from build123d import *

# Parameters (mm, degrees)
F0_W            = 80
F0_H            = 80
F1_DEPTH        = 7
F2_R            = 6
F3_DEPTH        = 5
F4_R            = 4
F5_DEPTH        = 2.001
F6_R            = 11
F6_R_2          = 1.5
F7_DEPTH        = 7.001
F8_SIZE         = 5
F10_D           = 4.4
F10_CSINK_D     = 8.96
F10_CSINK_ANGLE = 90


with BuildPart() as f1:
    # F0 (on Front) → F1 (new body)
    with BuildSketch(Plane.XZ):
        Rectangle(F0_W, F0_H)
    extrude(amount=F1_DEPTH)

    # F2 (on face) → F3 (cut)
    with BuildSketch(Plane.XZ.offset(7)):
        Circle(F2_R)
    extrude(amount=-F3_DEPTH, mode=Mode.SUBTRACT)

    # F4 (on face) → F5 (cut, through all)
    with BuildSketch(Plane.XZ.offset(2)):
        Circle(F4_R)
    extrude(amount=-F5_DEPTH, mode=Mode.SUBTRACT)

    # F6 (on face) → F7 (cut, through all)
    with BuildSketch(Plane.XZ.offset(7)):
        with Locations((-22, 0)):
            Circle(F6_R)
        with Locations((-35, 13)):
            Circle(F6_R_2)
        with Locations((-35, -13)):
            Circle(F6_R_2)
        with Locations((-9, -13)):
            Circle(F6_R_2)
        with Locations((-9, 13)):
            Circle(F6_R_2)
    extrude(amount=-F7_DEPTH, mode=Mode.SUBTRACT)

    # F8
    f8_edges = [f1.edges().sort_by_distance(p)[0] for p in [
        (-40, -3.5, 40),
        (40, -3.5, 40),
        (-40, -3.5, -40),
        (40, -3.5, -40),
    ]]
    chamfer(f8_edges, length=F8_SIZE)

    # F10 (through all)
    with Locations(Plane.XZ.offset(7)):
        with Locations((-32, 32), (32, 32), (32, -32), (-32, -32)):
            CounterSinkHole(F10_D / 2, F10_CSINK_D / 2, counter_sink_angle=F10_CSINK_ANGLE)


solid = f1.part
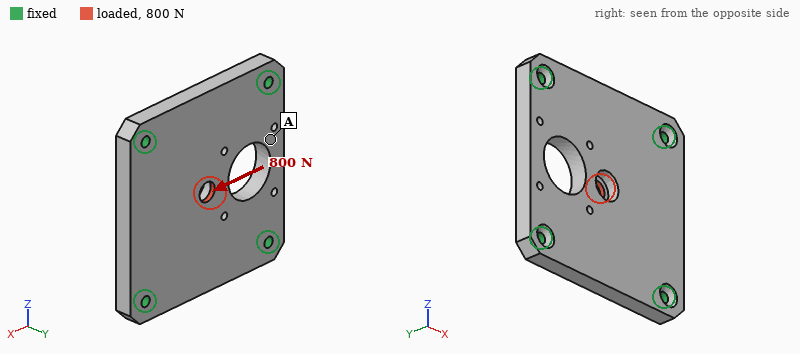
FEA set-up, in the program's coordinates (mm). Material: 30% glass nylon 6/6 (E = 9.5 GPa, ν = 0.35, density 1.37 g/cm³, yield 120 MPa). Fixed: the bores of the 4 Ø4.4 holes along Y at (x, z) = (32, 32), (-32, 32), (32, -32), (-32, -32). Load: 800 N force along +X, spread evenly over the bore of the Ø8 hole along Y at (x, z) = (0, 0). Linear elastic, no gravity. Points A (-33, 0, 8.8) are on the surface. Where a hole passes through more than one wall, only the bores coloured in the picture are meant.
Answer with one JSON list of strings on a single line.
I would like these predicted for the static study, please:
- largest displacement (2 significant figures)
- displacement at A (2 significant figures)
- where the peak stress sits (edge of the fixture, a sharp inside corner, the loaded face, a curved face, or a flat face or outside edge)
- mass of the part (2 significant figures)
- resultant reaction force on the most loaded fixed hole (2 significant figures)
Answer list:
["27 µm", "8.8 µm", "a sharp inside corner", "55 g", "230 N"]
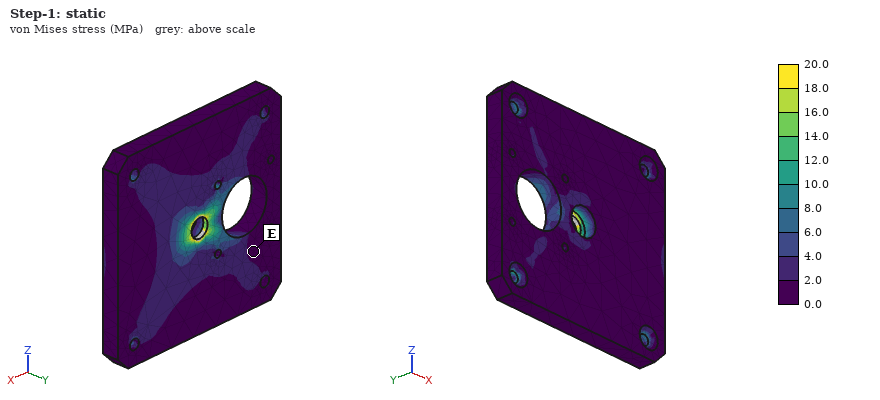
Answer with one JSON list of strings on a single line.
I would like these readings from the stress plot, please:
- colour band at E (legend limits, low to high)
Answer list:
["0.0 to 2.0 MPa"]
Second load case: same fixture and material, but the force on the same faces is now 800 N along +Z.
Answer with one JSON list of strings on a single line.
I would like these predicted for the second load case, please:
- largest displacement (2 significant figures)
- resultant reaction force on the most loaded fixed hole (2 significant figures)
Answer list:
["23 µm", "270 N"]
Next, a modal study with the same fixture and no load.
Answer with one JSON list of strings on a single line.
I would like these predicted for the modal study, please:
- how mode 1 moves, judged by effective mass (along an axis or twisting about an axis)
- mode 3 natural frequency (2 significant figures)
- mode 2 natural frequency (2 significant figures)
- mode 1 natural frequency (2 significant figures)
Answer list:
["along Y", "4300 Hz", "4100 Hz", "2600 Hz"]
